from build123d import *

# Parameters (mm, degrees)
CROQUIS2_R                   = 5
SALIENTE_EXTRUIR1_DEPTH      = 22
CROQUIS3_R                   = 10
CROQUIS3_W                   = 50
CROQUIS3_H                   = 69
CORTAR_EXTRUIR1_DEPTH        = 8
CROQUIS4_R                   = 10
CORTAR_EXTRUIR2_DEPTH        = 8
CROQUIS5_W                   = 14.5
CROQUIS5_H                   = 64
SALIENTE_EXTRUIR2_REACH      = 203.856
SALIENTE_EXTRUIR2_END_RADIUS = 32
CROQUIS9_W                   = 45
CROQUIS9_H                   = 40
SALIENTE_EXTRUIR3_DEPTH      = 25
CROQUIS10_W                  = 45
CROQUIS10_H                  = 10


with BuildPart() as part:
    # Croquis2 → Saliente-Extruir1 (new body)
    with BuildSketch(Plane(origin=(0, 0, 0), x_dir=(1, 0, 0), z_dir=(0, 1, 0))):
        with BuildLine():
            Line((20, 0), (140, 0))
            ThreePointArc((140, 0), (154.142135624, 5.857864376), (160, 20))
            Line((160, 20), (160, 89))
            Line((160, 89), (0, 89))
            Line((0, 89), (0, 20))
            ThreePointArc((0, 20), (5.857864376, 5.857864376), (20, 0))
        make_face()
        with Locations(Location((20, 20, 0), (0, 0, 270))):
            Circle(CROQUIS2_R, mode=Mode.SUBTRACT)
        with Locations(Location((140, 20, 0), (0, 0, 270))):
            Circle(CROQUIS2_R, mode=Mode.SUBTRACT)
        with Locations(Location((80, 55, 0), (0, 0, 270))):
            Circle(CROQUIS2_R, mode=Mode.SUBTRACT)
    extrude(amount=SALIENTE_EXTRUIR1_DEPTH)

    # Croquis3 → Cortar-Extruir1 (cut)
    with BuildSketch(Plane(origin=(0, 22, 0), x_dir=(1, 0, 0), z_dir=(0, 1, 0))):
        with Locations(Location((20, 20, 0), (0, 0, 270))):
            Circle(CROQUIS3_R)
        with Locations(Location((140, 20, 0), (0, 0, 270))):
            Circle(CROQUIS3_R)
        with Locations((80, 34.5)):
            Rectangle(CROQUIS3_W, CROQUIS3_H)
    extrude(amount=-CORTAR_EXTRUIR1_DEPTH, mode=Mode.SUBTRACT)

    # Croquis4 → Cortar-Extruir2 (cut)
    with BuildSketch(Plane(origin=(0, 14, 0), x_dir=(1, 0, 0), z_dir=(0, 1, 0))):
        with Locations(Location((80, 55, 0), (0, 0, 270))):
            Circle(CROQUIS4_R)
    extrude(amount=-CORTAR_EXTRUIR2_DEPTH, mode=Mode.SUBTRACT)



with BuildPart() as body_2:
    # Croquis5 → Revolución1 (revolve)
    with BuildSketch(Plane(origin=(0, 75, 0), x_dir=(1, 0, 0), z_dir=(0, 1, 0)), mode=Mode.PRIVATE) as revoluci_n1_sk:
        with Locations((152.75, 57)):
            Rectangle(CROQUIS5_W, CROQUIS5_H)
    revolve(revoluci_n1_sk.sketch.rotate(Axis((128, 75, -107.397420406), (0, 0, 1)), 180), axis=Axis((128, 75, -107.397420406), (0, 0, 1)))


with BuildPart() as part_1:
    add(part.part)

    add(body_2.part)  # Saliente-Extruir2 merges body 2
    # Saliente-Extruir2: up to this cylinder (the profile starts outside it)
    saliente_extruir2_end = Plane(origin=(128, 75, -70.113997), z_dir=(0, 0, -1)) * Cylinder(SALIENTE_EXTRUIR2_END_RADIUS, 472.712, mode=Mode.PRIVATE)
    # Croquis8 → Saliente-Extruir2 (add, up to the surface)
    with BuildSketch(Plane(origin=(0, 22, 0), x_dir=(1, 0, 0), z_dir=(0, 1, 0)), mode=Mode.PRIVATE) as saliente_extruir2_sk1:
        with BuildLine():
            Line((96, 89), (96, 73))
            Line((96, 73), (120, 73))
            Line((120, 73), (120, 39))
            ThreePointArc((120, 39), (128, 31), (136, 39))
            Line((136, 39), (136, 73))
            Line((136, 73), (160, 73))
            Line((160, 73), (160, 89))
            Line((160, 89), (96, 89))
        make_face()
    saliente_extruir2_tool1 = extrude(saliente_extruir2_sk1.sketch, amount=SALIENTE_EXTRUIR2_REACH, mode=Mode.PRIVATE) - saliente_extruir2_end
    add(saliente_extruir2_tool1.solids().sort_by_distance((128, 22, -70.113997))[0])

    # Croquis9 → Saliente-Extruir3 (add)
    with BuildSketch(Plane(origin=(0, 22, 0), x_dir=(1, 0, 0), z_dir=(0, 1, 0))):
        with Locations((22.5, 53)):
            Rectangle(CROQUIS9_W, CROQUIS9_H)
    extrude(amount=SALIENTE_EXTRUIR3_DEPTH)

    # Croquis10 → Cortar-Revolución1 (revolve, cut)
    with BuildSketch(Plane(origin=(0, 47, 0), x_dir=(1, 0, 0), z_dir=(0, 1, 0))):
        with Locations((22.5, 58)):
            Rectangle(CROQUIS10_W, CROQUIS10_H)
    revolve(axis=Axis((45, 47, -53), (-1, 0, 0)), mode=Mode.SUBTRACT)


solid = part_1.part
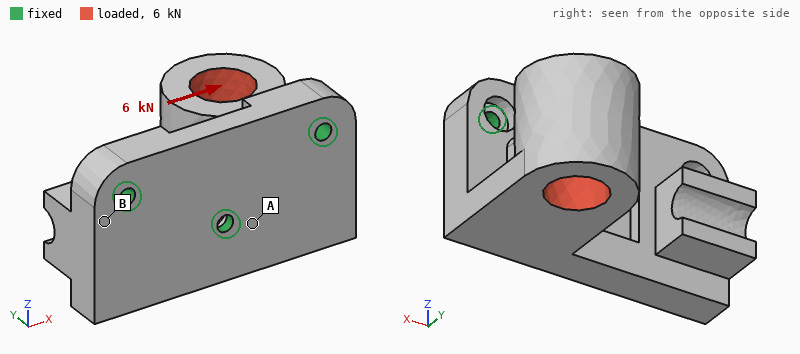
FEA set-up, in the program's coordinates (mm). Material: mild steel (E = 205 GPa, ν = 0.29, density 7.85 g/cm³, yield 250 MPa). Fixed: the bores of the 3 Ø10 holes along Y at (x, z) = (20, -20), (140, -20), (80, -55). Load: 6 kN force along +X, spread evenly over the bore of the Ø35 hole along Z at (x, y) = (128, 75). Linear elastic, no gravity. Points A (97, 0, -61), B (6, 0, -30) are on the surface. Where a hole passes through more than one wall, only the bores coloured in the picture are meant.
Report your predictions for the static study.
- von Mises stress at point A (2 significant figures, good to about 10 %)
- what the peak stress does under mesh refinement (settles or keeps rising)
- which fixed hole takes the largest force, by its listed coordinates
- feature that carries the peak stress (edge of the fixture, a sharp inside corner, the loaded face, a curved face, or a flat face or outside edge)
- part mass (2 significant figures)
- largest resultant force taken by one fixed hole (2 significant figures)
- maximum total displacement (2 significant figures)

28 MPa
keeps rising
(140, -20)
edge of the fixture
3.9 kg
5.8 kN
0.10 mm
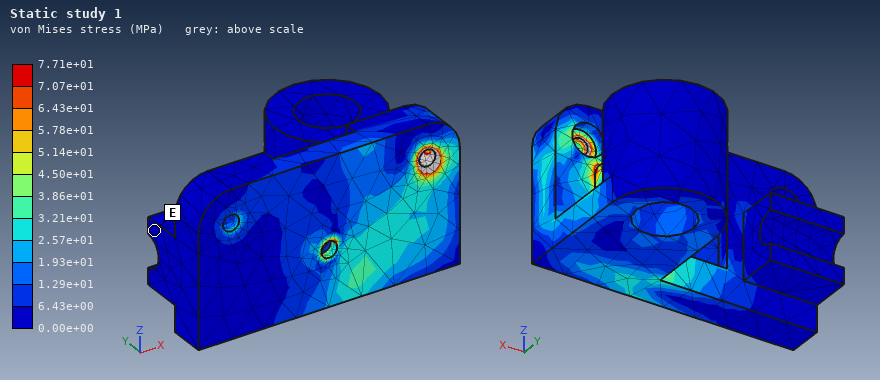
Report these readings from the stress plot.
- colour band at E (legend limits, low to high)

0.00e+00 to 6.43e+00 MPa
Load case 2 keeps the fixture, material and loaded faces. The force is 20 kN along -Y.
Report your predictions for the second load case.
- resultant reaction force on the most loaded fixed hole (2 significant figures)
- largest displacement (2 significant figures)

12 kN
0.14 mm
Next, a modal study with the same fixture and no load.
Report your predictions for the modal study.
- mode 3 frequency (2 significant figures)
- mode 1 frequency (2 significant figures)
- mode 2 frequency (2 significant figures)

3000 Hz
990 Hz
1800 Hz
